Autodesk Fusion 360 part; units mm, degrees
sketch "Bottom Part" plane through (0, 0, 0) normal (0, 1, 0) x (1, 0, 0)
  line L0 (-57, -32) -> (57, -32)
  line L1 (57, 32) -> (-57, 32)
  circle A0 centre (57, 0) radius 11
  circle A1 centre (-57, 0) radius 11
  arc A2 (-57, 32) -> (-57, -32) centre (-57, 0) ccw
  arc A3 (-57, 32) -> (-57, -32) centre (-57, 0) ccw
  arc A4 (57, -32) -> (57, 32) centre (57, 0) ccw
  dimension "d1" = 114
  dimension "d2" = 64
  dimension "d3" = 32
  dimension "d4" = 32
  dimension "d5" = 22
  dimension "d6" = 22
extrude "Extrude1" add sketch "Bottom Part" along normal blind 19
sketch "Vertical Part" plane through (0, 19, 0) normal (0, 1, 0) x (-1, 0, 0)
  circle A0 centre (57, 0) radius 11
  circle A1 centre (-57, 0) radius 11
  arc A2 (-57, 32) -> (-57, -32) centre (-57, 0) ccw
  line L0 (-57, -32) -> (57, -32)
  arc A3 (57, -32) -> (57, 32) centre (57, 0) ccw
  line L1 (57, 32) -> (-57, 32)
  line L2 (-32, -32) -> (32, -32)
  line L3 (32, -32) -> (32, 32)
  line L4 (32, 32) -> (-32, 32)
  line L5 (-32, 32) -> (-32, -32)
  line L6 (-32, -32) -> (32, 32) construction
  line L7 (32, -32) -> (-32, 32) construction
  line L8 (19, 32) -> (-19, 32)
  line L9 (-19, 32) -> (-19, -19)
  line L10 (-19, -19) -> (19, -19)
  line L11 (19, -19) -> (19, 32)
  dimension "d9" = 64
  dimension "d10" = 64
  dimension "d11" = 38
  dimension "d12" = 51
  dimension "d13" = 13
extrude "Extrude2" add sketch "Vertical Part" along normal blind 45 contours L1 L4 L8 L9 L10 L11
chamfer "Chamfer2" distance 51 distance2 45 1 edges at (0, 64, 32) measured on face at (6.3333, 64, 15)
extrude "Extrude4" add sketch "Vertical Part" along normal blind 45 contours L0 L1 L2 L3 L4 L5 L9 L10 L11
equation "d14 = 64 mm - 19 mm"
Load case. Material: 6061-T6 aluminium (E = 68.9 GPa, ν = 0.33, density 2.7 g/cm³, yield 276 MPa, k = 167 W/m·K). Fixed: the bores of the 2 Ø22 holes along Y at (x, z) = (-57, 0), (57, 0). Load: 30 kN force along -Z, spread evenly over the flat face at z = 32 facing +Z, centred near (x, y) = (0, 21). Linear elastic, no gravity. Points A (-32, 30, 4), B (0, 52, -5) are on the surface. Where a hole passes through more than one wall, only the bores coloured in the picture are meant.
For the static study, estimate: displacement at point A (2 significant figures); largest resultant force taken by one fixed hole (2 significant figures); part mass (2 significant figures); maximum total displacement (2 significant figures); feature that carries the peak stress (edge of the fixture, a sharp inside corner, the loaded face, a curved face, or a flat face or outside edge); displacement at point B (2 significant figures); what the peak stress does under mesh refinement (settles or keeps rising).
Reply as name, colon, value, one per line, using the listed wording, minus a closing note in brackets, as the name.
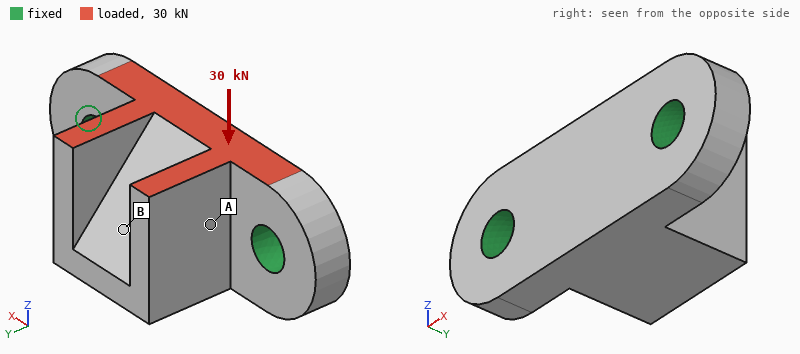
displacement at point A: 38 µm
largest resultant force taken by one fixed hole: 15 kN
part mass: 880 g
maximum total displacement: 89 µm
feature that carries the peak stress: edge of the fixture
displacement at point B: 62 µm
what the peak stress does under mesh refinement: keeps rising
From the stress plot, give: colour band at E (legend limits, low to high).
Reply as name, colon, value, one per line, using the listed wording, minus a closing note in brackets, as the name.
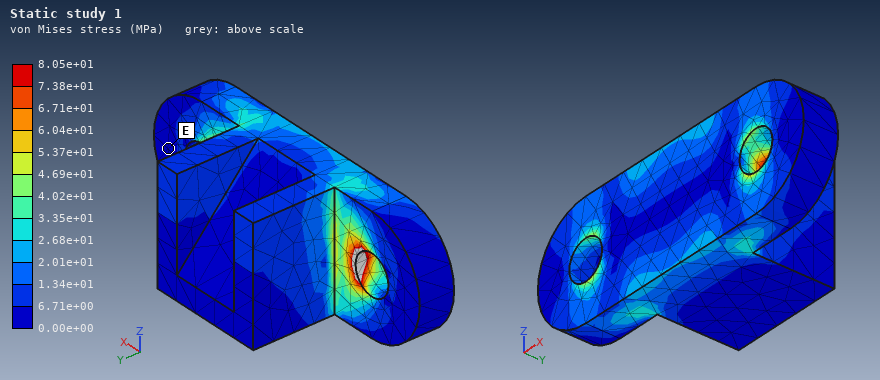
colour band at E: 0.00e+00 to 6.71e+00 MPa
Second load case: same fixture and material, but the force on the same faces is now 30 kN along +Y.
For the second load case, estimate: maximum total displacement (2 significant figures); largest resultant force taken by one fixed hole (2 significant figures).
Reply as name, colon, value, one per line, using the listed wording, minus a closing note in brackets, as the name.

maximum total displacement: 0.18 mm
largest resultant force taken by one fixed hole: 16 kN
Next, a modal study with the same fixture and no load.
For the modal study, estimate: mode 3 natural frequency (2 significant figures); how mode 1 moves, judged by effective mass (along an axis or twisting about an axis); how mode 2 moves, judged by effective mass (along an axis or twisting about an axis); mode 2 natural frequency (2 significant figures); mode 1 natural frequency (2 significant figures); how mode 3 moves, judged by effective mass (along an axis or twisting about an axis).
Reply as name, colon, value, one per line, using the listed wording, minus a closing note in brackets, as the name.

mode 3 natural frequency: 7100 Hz
how mode 1 moves, judged by effective mass: along Z
how mode 2 moves, judged by effective mass: along Y
mode 2 natural frequency: 6300 Hz
mode 1 natural frequency: 3500 Hz
how mode 3 moves, judged by effective mass: along X
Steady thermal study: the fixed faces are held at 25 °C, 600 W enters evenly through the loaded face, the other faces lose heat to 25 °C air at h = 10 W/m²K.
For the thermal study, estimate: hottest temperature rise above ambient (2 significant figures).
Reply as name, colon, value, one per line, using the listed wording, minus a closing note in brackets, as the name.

hottest temperature rise above ambient: 71 K
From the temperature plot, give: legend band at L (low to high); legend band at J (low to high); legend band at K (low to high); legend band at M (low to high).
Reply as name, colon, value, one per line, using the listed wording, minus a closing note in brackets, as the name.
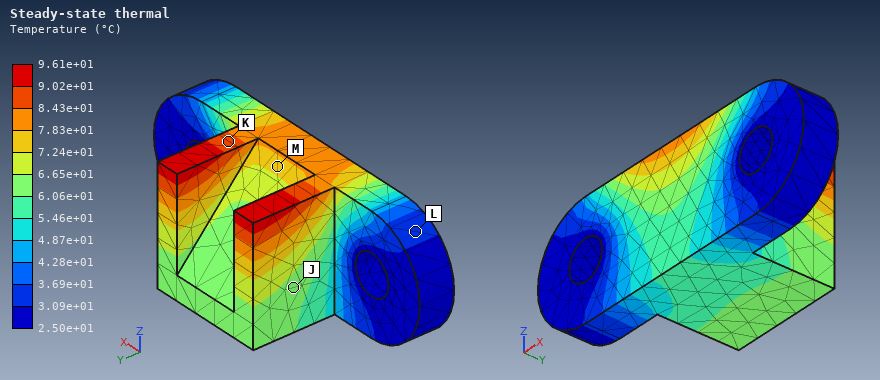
legend band at L: 3.09e+01 to 3.69e+01 °C
legend band at J: 6.06e+01 to 6.65e+01 °C
legend band at K: 8.43e+01 to 9.02e+01 °C
legend band at M: 7.24e+01 to 7.83e+01 °C
